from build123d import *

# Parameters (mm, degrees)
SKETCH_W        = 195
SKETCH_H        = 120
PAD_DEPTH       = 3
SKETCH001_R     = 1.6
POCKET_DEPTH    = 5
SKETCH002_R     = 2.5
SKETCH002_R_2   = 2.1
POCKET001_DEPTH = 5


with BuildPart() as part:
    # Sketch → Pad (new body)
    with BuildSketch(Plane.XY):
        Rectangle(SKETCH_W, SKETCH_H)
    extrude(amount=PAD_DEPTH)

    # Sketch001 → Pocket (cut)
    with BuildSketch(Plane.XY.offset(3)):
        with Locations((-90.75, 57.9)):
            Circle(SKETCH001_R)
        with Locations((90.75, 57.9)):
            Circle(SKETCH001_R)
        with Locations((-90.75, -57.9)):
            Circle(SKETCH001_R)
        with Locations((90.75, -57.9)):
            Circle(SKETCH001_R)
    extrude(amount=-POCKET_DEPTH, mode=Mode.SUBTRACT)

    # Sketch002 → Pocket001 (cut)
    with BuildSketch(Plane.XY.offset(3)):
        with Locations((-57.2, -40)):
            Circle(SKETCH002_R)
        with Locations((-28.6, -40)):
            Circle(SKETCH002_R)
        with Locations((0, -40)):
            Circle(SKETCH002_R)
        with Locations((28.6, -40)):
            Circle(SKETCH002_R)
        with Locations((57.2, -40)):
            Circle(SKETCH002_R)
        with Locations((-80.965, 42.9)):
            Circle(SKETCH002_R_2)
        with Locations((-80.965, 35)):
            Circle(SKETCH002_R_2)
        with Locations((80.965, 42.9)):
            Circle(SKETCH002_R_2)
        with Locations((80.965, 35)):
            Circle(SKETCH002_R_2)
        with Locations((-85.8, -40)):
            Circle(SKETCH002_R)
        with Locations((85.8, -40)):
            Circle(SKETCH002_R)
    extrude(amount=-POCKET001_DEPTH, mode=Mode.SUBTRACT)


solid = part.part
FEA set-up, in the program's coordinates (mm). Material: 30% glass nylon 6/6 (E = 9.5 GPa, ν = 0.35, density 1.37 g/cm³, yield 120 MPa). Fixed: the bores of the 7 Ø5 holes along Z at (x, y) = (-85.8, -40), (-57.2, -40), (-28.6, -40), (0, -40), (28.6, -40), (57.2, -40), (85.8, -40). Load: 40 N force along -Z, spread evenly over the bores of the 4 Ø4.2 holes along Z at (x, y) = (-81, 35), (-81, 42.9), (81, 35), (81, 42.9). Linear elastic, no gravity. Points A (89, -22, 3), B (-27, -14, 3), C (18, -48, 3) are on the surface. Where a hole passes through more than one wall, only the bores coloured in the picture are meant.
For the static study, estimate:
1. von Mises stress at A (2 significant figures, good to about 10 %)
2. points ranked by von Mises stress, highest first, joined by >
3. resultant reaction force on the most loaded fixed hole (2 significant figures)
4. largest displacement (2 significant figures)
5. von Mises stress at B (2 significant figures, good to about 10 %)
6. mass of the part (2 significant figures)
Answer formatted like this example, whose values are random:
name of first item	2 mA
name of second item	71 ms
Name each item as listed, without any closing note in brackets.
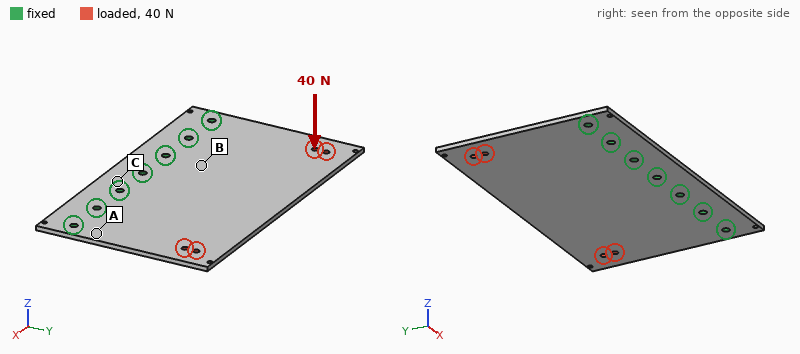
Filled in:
von Mises stress at A	9.0 MPa
points ranked by von Mises stress, highest first, joined by >	A > B > C
resultant reaction force on the most loaded fixed hole	8.4 N
largest displacement	2.4 mm
von Mises stress at B	5.9 MPa
mass of the part	95 g
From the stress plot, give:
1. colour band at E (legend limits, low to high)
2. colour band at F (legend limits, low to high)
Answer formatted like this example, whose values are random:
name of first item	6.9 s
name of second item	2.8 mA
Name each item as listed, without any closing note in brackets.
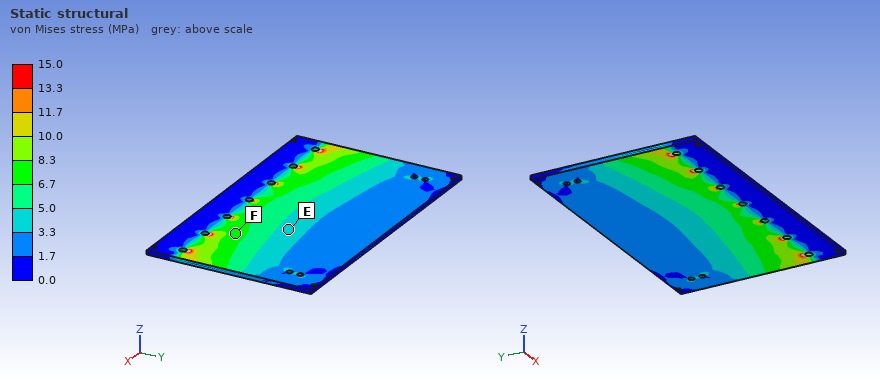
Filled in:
colour band at E	3.3 to 5.0 MPa
colour band at F	6.7 to 8.3 MPa
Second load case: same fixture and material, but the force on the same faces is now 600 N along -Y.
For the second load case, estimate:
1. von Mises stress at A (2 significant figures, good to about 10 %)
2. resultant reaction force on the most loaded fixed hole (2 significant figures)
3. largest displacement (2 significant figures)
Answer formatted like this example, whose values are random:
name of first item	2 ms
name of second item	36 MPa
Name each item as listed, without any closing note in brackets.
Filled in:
von Mises stress at A	2.1 MPa
resultant reaction force on the most loaded fixed hole	140 N
largest displacement	23 µm
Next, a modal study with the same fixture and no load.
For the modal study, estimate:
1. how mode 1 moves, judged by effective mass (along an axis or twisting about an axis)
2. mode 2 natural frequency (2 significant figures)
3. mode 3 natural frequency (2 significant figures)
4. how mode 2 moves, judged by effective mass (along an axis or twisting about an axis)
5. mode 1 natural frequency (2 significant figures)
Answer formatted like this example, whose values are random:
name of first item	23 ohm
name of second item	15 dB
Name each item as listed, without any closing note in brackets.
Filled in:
how mode 1 moves, judged by effective mass	along Z
mode 2 natural frequency	210 Hz
mode 3 natural frequency	400 Hz
how mode 2 moves, judged by effective mass	twisting about Y
mode 1 natural frequency	130 Hz
